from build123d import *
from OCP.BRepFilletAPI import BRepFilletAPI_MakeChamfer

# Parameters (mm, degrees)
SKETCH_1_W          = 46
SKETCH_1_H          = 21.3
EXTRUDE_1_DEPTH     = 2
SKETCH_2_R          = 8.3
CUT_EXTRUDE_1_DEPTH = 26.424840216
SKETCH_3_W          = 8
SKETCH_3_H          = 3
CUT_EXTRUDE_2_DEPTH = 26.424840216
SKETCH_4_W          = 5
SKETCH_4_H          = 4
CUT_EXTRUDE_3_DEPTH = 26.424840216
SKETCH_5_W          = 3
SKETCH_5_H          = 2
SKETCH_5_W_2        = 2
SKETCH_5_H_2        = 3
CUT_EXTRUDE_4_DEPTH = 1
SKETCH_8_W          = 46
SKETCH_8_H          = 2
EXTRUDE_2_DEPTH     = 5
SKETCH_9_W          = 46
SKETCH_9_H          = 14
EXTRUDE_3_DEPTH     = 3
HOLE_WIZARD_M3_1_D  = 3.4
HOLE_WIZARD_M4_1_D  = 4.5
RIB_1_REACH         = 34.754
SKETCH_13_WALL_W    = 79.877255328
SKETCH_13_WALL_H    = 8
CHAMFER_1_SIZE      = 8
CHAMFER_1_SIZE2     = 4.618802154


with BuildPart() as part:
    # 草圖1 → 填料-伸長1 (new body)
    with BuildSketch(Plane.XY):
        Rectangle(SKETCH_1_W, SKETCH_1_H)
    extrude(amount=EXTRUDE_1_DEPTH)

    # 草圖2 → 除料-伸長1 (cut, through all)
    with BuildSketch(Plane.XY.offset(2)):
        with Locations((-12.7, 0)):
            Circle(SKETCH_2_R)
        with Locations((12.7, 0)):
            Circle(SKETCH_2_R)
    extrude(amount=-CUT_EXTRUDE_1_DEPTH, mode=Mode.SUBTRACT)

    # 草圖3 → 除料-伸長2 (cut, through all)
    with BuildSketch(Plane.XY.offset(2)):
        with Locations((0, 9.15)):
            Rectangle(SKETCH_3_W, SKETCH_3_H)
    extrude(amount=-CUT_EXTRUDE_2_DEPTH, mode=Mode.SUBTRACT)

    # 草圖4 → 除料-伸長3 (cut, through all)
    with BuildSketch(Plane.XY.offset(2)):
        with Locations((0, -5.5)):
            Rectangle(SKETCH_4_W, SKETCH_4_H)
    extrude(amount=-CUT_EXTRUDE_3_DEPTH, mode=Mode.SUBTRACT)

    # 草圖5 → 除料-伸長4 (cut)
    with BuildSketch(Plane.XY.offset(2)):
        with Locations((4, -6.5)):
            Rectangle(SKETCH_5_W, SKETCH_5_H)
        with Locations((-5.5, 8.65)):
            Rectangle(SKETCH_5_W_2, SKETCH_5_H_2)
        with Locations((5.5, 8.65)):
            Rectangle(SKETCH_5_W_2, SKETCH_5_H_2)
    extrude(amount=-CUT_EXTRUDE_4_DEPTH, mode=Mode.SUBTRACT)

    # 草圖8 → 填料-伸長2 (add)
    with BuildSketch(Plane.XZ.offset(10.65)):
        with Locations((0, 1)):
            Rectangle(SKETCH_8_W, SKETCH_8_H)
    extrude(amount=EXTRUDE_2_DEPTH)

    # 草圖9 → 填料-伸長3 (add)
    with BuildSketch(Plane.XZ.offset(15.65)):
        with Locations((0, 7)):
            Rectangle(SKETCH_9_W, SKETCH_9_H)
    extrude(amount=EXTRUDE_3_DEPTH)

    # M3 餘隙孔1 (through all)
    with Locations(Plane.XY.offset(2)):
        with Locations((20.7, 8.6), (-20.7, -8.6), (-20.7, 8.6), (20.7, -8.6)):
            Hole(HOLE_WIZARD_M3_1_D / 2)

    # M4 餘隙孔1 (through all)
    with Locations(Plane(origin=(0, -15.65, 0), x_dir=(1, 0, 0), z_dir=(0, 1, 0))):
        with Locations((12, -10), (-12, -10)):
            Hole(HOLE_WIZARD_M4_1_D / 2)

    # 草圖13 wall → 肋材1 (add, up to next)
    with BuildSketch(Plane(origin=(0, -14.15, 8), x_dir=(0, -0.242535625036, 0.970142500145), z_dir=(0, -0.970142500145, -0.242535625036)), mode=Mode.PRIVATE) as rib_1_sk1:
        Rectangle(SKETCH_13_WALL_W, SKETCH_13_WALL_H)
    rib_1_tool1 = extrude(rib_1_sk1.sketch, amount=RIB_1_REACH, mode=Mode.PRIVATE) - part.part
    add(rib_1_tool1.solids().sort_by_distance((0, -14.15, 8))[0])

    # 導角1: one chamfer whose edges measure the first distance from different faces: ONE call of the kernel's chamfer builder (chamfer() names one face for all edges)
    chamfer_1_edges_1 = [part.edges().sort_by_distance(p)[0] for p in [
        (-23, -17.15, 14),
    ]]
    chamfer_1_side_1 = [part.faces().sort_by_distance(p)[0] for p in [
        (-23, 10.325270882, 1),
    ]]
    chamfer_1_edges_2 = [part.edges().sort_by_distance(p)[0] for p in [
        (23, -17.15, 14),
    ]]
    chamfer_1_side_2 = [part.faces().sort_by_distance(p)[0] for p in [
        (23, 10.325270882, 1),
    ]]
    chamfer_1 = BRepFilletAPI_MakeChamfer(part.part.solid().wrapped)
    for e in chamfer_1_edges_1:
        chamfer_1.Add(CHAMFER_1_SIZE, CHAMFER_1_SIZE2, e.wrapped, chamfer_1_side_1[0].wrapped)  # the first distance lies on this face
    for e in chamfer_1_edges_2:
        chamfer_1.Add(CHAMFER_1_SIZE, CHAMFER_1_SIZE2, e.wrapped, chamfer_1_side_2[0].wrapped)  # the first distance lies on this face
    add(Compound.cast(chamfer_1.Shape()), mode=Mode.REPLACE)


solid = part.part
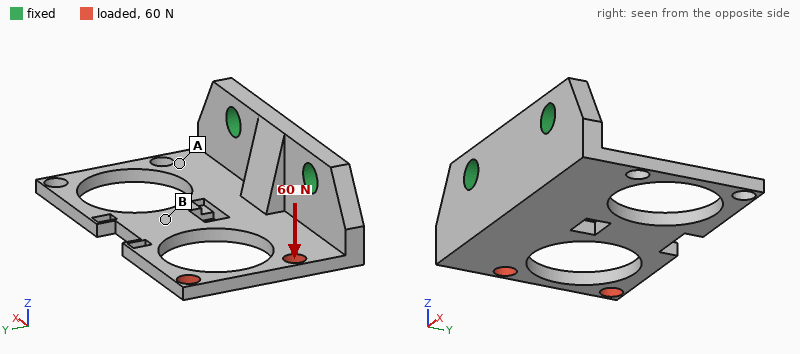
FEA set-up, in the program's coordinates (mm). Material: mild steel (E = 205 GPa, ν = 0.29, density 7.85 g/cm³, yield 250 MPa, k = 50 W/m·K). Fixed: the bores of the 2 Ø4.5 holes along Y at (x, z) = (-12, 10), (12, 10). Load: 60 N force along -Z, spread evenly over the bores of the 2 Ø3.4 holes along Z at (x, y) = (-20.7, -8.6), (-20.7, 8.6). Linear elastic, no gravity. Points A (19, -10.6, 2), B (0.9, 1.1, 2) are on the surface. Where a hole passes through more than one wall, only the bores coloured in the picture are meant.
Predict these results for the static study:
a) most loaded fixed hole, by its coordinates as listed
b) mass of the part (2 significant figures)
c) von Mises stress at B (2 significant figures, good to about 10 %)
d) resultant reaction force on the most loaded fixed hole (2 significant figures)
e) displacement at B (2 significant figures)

(-12, 10)
25 g
32 MPa
70 N
0.025 mm
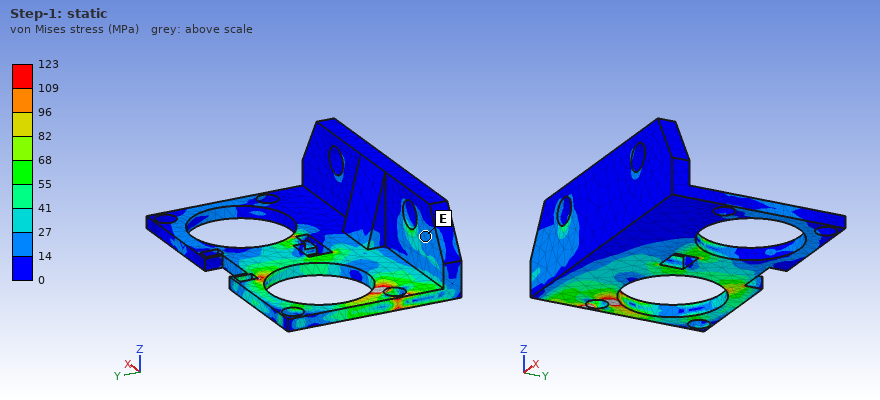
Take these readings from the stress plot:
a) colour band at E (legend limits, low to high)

14 to 27 MPa
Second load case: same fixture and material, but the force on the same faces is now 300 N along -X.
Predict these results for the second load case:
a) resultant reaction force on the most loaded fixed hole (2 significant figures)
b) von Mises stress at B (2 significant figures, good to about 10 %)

270 N
20 MPa
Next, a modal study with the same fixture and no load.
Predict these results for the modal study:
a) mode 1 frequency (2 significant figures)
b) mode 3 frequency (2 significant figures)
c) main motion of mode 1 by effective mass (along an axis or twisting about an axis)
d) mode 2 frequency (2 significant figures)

2200 Hz
6000 Hz
along Z
3400 Hz
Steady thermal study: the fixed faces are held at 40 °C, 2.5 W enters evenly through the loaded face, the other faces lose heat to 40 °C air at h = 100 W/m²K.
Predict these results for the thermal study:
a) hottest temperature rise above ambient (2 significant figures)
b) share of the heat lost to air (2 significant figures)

41 K
55 %
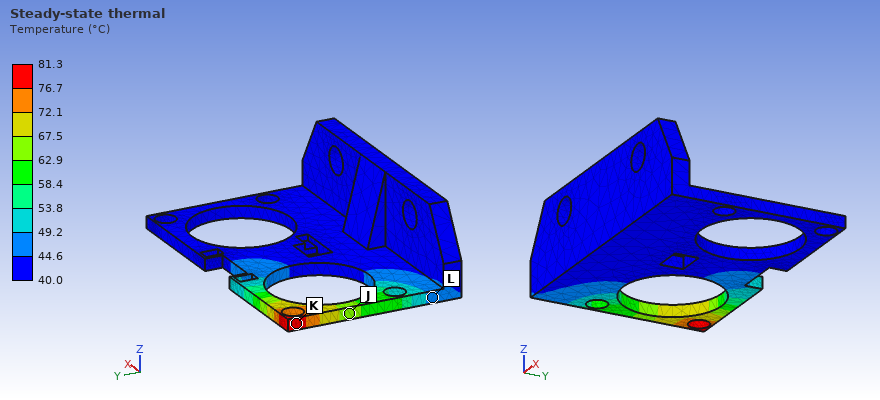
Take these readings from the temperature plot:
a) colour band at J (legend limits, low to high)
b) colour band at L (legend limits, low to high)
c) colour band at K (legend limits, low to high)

62.9 to 67.5 °C
44.6 to 49.2 °C
76.7 to 81.3 °C
